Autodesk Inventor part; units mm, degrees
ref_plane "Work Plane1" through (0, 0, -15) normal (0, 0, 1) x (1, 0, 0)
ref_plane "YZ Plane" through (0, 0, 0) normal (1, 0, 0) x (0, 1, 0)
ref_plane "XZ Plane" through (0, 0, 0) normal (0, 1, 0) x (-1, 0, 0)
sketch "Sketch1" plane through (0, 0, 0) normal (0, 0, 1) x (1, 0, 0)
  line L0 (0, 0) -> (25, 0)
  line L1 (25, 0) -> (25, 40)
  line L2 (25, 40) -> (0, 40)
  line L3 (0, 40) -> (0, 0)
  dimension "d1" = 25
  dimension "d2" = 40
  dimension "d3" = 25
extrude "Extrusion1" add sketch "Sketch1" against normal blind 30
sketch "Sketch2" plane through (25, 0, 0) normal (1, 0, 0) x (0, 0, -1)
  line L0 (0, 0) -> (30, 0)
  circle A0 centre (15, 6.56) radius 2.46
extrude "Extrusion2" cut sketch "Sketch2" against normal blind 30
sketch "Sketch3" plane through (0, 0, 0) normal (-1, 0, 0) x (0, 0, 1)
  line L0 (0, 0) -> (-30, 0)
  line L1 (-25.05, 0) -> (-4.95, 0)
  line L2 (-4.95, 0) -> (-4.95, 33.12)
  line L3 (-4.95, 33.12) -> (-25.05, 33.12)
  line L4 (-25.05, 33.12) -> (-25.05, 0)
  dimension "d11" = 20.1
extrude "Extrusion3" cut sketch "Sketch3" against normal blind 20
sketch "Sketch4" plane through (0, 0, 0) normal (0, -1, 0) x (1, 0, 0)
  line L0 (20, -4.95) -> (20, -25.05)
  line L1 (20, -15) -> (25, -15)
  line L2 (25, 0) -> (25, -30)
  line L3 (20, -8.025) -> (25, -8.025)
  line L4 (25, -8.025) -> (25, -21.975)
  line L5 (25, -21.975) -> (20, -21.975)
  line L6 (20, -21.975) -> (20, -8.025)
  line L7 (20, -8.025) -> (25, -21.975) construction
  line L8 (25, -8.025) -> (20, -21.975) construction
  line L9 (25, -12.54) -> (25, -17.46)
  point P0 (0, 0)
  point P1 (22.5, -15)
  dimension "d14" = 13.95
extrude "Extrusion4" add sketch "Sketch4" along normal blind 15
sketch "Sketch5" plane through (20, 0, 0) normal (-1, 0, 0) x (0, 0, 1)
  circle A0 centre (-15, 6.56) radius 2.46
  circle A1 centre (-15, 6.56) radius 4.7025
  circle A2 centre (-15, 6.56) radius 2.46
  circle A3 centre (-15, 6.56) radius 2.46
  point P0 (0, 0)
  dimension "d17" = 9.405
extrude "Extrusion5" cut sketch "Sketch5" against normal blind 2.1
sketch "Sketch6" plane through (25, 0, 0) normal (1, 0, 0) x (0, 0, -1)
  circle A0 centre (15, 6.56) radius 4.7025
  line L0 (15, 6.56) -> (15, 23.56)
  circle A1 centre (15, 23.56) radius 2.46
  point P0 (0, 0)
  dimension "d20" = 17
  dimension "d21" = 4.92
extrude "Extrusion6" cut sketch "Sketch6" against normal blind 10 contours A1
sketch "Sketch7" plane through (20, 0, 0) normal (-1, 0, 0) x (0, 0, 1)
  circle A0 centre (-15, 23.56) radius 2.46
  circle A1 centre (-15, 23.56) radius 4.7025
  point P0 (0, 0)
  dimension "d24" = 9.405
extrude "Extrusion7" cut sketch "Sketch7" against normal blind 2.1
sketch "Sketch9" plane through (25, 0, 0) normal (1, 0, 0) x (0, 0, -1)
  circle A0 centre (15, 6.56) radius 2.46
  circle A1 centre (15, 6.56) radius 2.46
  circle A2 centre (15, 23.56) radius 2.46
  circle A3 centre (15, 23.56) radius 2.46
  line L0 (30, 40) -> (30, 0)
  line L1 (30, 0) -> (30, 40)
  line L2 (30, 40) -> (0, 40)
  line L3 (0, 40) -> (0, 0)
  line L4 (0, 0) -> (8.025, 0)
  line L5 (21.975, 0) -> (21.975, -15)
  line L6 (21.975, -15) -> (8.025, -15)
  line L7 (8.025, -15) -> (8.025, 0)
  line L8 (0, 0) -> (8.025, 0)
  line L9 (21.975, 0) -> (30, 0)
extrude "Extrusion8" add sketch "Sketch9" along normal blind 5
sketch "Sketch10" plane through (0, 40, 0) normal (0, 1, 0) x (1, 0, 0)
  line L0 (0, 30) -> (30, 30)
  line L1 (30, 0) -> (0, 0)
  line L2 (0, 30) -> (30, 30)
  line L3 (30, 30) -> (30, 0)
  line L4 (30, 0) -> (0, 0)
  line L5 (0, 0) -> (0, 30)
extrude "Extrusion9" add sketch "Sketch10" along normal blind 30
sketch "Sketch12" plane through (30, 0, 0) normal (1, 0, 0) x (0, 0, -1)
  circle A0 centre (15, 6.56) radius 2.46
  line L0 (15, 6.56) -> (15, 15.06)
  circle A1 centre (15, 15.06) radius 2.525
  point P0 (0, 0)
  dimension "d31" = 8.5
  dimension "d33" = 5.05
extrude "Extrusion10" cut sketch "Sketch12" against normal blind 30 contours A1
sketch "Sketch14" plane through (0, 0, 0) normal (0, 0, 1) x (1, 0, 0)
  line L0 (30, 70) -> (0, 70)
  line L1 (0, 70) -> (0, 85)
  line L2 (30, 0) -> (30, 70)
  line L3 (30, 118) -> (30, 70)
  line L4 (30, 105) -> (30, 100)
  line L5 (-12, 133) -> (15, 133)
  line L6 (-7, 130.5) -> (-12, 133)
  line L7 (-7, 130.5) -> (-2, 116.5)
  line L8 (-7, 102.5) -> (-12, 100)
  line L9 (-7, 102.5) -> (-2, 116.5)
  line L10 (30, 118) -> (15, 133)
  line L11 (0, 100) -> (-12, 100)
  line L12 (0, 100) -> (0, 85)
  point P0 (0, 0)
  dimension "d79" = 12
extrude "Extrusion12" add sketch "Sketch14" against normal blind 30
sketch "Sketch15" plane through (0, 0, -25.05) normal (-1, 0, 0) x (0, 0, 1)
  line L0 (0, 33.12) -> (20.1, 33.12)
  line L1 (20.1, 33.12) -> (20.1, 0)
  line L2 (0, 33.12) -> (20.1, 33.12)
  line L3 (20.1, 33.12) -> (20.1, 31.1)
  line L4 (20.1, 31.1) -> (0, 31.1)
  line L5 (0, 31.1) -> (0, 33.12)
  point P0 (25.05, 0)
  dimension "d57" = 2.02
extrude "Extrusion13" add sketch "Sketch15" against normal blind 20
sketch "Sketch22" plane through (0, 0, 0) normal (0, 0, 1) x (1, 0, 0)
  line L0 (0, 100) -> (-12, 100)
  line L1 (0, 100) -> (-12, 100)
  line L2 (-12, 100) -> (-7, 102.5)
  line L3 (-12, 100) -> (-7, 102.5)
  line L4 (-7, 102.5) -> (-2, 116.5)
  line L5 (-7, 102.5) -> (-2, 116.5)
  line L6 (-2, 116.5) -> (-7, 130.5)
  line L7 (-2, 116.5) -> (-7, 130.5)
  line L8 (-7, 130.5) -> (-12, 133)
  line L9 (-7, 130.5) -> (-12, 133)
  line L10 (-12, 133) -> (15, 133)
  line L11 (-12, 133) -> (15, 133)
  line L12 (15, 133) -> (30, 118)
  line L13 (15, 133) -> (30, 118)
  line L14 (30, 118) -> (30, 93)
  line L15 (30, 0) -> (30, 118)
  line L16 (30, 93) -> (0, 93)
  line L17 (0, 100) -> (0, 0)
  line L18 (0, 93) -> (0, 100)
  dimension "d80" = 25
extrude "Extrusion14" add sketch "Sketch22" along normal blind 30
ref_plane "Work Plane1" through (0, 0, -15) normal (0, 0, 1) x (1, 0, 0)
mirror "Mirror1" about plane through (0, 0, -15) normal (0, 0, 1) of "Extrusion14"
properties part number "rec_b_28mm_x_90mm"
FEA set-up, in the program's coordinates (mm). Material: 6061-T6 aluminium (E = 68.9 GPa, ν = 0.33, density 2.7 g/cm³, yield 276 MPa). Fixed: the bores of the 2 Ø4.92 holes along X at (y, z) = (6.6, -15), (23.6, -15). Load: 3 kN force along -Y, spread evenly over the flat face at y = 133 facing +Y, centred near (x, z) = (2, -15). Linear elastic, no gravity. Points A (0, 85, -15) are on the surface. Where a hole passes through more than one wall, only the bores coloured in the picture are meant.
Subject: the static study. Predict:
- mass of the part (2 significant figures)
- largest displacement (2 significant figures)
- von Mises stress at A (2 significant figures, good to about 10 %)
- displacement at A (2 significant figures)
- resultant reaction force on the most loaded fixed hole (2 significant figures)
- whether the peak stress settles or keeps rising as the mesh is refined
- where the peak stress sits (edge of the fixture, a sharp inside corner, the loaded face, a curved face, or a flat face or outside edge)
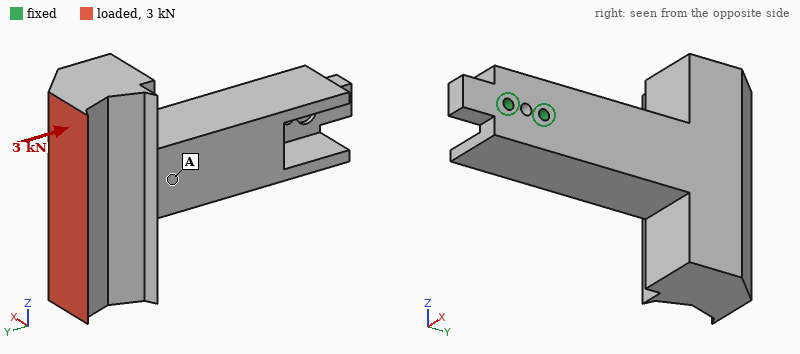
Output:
500 g
0.23 mm
11 MPa
0.12 mm
3.4 kN
keeps rising
edge of the fixture
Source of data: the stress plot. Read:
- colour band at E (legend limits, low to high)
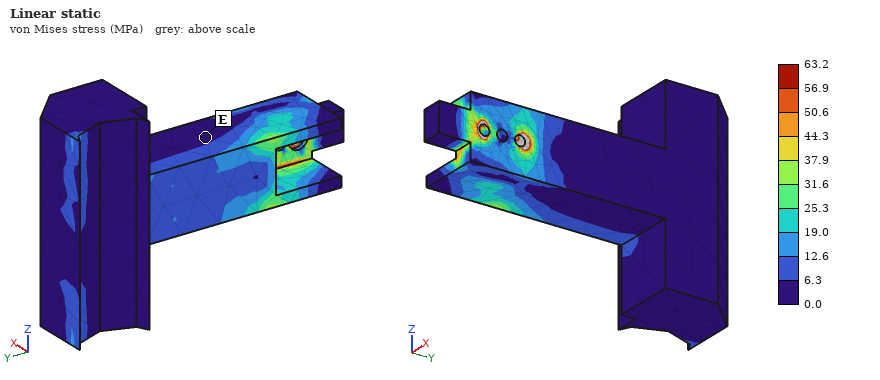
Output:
0.0 to 6.3 MPa
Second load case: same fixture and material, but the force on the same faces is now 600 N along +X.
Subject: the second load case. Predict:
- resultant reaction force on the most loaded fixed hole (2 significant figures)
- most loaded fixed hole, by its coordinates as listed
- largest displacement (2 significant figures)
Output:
3.2 kN
(23.6, -15)
0.22 mm
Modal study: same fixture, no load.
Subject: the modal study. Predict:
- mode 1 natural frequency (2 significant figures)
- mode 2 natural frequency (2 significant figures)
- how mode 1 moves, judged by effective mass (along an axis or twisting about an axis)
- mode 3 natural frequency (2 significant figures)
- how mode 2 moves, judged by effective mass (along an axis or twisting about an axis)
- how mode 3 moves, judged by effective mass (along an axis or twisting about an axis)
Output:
570 Hz
640 Hz
along X
1200 Hz
along Z
twisting about Y
